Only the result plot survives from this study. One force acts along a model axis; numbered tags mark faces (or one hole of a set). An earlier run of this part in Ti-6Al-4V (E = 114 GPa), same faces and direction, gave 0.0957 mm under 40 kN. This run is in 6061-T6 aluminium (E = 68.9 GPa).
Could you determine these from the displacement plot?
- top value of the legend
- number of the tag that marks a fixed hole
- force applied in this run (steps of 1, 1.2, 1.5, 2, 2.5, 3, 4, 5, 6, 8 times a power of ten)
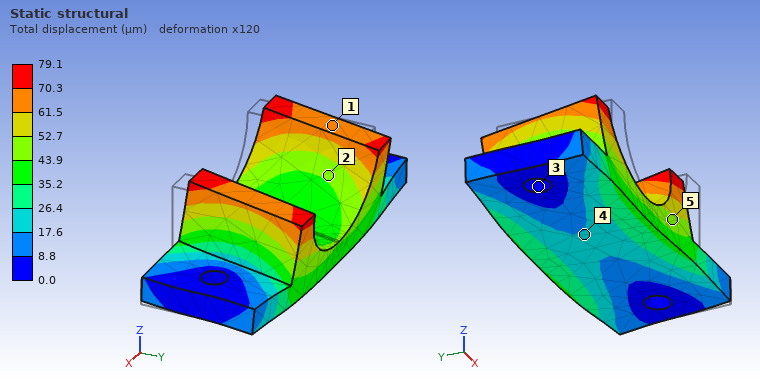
79.1 µm
3
20 kN
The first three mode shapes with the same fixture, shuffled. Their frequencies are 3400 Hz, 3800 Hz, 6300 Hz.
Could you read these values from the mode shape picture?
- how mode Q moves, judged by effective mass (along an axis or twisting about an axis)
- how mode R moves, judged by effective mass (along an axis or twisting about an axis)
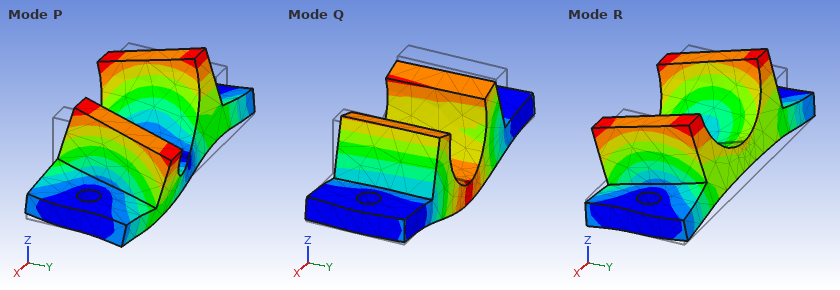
along Z
along Y
